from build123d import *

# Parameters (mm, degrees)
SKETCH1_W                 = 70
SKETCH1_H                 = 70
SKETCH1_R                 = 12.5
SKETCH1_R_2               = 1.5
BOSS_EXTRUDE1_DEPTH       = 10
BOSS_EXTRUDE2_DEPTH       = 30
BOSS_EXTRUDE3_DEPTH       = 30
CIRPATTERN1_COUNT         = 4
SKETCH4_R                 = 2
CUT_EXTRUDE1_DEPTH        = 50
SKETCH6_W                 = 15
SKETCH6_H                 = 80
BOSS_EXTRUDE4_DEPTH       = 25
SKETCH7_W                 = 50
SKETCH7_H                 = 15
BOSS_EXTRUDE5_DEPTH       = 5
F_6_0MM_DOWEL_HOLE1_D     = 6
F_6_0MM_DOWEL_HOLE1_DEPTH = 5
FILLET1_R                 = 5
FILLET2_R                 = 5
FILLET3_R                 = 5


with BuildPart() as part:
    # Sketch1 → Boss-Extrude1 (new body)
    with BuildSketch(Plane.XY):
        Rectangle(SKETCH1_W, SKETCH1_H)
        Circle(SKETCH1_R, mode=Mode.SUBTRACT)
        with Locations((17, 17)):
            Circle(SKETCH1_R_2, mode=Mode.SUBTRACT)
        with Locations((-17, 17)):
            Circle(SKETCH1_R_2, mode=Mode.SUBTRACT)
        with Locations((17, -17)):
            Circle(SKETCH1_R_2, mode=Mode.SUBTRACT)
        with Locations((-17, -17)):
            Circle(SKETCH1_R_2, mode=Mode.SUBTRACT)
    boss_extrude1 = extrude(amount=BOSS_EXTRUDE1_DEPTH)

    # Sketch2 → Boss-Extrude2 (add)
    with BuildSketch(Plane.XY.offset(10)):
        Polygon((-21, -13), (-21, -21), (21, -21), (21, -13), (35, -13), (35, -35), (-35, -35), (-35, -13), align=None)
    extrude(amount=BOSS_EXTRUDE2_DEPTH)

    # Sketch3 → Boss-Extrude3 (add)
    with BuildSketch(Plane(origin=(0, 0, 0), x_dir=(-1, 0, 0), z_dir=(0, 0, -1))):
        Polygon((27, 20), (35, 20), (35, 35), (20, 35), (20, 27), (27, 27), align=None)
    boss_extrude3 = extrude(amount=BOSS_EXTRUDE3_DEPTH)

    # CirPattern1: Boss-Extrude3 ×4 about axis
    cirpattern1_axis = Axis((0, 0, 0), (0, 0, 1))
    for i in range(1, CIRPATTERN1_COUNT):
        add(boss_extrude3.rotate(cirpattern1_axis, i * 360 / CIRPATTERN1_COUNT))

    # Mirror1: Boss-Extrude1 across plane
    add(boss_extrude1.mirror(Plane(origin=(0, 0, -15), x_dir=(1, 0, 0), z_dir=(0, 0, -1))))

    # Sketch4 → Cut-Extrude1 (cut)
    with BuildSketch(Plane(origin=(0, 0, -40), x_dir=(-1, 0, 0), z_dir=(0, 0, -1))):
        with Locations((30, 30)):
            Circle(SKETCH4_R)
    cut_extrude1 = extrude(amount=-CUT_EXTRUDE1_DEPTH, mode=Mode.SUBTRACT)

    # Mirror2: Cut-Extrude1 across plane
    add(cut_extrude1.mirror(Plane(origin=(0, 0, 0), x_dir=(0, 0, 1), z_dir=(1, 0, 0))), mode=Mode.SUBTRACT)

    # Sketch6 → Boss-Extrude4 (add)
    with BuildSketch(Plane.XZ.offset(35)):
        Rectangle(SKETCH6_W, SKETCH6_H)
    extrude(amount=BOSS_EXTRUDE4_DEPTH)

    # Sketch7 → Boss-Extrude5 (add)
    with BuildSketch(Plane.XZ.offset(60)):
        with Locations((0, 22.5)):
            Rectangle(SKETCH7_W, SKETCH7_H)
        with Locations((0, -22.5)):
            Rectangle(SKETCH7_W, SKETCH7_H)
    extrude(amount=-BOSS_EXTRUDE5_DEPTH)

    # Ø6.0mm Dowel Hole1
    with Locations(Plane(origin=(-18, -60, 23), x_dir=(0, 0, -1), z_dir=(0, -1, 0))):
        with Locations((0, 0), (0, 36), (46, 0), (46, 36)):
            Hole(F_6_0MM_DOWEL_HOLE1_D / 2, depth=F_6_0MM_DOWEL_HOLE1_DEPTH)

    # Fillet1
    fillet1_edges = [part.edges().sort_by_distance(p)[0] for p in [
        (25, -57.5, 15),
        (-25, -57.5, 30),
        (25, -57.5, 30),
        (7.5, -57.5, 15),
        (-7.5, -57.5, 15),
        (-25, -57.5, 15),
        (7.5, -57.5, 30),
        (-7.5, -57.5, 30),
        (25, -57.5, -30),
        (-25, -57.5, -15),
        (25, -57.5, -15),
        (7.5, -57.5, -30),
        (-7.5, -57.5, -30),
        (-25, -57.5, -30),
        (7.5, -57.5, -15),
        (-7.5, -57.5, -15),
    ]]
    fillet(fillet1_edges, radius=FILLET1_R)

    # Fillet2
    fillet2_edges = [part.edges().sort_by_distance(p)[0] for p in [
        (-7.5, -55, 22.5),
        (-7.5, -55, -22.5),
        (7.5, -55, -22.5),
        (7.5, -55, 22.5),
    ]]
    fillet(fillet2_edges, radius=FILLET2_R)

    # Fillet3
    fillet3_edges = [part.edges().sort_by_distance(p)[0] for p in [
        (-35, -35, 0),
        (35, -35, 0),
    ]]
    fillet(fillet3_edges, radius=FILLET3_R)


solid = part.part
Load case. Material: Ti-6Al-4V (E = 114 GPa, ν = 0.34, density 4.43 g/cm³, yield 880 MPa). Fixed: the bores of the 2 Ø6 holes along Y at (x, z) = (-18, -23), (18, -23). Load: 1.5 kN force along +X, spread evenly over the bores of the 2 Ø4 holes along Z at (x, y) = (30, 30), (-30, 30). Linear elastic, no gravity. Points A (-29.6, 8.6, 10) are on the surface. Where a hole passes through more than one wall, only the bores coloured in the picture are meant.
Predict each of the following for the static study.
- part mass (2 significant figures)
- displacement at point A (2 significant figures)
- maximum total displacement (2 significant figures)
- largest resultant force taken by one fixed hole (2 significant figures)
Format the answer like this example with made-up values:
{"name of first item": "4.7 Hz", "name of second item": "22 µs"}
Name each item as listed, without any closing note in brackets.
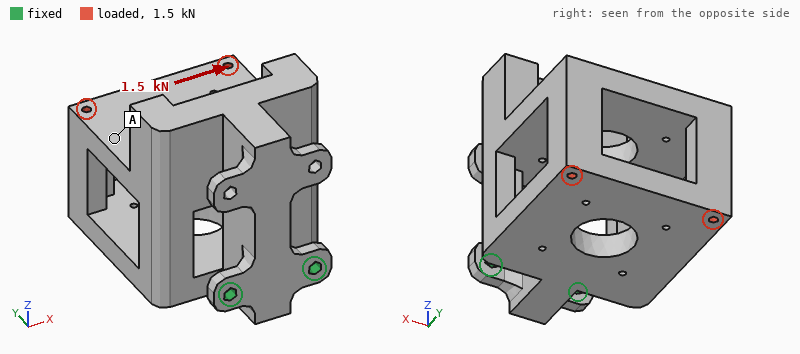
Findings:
{"part mass": "790 g", "displacement at point A": "0.37 mm", "maximum total displacement": "0.52 mm", "largest resultant force taken by one fixed hole": "5.0 kN"}
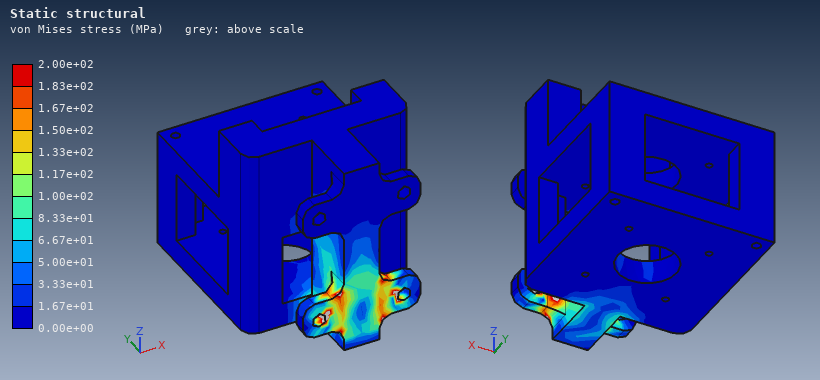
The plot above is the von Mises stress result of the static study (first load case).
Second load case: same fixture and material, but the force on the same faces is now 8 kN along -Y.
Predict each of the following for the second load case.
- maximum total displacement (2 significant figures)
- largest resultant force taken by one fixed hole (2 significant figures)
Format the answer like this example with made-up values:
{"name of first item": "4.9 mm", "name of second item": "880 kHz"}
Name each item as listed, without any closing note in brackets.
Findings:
{"maximum total displacement": "0.82 mm", "largest resultant force taken by one fixed hole": "4.6 kN"}
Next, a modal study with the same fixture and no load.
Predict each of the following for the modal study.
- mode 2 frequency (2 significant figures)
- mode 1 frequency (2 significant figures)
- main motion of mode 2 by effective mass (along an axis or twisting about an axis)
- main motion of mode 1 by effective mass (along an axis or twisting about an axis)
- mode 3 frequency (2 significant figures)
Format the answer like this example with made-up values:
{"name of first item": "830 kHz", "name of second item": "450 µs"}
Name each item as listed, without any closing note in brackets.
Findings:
{"mode 2 frequency": "540 Hz", "mode 1 frequency": "260 Hz", "main motion of mode 2 by effective mass": "along X", "main motion of mode 1 by effective mass": "along Z", "mode 3 frequency": "1200 Hz"}
